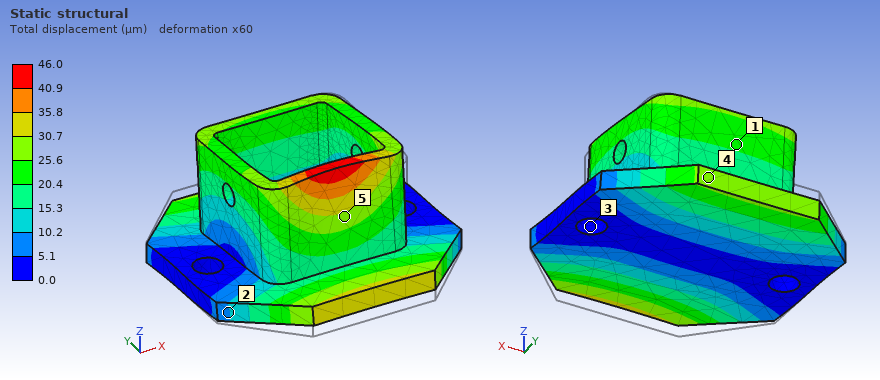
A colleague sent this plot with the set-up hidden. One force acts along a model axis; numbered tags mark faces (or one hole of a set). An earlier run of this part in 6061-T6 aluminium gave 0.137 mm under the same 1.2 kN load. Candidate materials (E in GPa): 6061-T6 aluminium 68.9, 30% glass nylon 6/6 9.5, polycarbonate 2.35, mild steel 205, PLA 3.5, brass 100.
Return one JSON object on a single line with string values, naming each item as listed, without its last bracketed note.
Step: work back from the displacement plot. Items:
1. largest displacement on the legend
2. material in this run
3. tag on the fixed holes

{"largest displacement on the legend": "46.0 µm", "material in this run": "mild steel", "tag on the fixed holes": "3"}
